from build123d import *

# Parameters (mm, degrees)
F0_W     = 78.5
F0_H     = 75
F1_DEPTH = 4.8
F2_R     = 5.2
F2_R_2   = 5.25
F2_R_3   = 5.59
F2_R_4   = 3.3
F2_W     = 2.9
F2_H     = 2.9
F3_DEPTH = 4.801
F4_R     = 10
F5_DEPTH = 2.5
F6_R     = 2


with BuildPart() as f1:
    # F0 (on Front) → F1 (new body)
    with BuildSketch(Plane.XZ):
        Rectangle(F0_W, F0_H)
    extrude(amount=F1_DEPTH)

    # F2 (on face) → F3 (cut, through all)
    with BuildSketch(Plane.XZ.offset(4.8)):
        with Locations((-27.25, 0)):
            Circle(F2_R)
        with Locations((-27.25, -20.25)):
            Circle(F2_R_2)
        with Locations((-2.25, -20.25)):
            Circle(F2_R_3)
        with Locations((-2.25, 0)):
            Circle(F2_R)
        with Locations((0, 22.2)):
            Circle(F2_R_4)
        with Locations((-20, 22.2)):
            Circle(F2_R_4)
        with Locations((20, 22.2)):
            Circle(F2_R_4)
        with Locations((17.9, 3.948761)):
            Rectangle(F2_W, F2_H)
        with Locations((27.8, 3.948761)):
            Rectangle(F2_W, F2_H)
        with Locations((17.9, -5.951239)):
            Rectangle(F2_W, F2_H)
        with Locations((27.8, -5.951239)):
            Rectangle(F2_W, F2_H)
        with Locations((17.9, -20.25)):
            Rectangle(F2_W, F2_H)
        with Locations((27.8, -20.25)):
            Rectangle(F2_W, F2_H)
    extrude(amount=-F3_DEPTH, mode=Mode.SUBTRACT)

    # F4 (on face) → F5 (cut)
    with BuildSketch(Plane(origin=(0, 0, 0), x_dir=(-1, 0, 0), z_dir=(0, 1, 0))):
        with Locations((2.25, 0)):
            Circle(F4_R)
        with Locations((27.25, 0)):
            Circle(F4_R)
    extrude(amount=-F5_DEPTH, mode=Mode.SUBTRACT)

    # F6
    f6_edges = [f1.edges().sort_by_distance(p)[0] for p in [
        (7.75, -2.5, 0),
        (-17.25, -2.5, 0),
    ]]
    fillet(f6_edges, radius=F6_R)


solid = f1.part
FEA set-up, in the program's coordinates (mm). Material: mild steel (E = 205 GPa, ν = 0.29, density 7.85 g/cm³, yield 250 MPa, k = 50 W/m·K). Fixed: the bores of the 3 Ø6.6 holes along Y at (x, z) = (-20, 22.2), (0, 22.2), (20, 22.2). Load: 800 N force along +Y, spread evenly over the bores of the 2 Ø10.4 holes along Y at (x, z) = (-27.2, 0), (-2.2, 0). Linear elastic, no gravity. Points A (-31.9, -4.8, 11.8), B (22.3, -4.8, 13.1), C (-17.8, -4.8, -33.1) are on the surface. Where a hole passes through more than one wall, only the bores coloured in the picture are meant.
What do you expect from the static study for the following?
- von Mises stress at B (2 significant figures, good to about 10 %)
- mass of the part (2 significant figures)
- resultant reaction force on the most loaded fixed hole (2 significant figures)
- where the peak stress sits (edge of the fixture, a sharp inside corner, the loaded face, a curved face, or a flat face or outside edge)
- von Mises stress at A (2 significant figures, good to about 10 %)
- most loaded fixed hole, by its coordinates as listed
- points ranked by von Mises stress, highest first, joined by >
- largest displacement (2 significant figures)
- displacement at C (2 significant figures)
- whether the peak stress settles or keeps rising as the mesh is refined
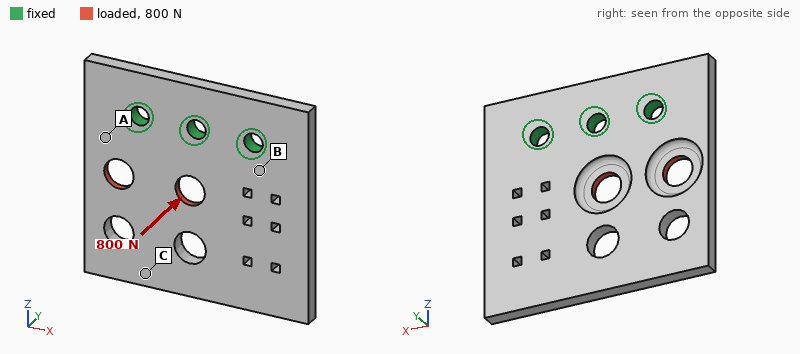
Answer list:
24 MPa
190 g
500 N
edge of the fixture
38 MPa
(-20, 22.2)
A > B > C
97 µm
77 µm
keeps rising
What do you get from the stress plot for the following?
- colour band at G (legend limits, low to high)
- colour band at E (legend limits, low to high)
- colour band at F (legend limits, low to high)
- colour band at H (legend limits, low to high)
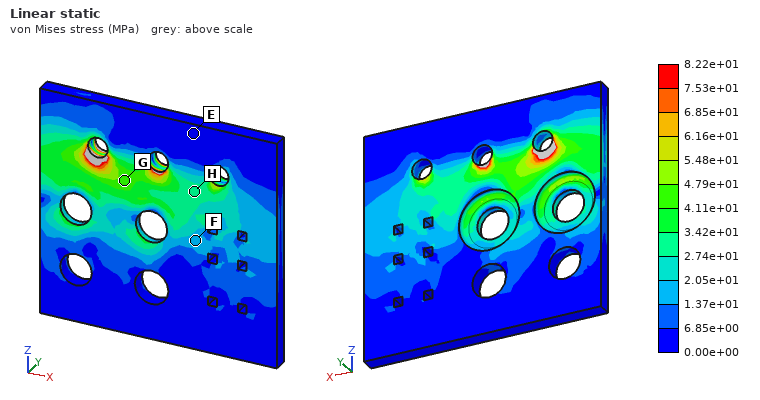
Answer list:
4.11e+01 to 4.79e+01 MPa
0.00e+00 to 6.85e+00 MPa
1.37e+01 to 2.05e+01 MPa
2.74e+01 to 3.42e+01 MPa
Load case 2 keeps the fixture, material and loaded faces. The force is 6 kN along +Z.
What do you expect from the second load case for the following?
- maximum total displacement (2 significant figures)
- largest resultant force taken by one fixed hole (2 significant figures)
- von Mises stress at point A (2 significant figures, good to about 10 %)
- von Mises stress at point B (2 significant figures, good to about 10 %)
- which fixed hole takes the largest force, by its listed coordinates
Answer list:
65 µm
4.2 kN
56 MPa
17 MPa
(-20, 22.2)
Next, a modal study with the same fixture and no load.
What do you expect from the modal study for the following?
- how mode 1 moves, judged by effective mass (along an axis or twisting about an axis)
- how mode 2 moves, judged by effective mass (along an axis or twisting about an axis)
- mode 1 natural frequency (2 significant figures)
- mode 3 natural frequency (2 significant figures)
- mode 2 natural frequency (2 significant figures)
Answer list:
along Y
twisting about Z
1000 Hz
4800 Hz
2000 Hz
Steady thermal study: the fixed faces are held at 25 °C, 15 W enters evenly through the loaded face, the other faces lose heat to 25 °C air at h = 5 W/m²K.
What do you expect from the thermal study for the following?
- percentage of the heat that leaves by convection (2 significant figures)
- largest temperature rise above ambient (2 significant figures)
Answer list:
6.0 %
37 K
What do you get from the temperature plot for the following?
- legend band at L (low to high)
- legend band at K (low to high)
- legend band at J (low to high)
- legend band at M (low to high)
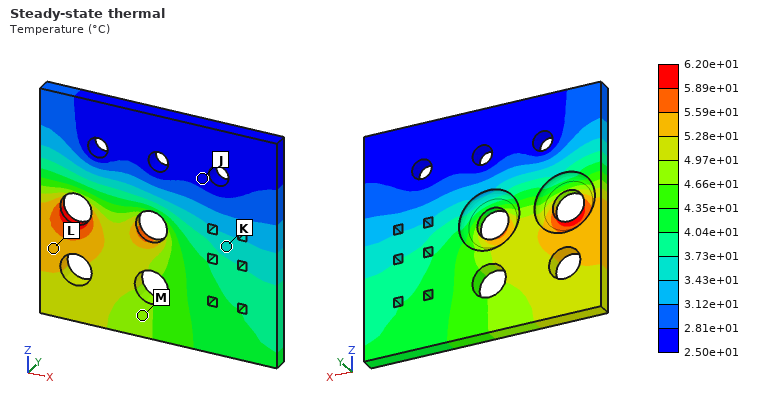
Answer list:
5.28e+01 to 5.59e+01 °C
3.43e+01 to 3.73e+01 °C
2.50e+01 to 2.81e+01 °C
4.66e+01 to 4.97e+01 °C
